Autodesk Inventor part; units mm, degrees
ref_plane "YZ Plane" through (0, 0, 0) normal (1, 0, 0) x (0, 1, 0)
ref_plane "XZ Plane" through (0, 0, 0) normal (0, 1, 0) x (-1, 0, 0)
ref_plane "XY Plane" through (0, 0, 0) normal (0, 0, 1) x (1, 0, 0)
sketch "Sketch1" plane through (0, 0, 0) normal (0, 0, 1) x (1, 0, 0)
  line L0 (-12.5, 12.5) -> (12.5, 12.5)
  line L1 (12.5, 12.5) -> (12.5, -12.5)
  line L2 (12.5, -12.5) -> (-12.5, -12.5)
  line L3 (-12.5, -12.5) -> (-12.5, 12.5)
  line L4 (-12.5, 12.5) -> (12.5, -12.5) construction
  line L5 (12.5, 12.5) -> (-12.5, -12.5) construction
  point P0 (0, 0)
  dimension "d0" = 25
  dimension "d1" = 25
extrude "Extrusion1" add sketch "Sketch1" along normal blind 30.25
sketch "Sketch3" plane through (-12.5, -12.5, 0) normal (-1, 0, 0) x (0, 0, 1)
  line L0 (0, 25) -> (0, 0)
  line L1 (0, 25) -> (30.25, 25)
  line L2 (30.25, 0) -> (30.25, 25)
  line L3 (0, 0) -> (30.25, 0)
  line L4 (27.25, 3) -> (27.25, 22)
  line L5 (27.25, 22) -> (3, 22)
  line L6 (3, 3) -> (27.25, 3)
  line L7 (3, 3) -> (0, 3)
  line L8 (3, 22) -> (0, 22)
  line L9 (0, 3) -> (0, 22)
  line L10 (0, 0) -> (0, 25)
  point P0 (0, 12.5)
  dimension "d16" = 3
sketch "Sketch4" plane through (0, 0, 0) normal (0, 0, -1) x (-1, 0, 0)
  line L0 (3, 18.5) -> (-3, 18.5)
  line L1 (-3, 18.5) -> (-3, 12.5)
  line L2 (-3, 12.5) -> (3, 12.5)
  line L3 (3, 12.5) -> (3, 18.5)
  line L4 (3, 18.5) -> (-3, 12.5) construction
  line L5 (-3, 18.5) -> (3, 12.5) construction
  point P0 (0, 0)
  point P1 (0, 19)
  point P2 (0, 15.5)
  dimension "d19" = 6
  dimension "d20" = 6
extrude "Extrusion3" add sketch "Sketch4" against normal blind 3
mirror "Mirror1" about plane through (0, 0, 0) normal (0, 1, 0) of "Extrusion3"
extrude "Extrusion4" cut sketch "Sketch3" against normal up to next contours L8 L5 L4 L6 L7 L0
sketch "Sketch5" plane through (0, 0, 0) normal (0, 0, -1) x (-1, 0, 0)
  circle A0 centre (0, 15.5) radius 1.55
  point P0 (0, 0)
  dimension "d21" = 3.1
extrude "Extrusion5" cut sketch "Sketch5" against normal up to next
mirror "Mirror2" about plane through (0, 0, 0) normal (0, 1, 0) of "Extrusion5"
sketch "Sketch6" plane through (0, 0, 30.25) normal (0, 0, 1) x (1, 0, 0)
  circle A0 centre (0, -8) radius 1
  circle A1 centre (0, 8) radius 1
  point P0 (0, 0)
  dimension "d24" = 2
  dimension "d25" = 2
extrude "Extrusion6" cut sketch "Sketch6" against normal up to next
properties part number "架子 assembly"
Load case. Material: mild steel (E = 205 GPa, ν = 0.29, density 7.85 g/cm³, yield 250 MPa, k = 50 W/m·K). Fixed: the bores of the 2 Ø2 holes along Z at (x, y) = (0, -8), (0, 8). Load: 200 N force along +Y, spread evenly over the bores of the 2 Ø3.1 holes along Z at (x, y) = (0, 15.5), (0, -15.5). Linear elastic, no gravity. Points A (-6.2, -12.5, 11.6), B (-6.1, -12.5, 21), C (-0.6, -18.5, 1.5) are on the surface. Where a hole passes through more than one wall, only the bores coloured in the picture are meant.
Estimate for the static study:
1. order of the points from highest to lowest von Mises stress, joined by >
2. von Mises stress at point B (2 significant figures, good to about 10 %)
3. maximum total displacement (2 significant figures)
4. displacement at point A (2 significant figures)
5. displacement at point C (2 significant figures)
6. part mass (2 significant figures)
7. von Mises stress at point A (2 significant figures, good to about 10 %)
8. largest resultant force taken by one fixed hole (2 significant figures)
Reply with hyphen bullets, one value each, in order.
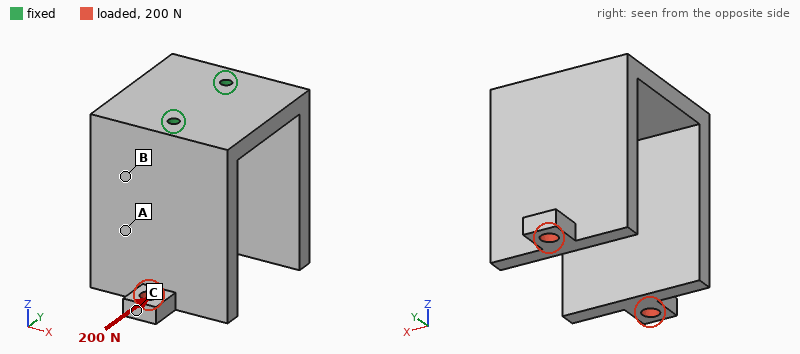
- B > A > C
- 48 MPa
- 90 µm
- 40 µm
- 84 µm
- 48 g
- 27 MPa
- 200 N
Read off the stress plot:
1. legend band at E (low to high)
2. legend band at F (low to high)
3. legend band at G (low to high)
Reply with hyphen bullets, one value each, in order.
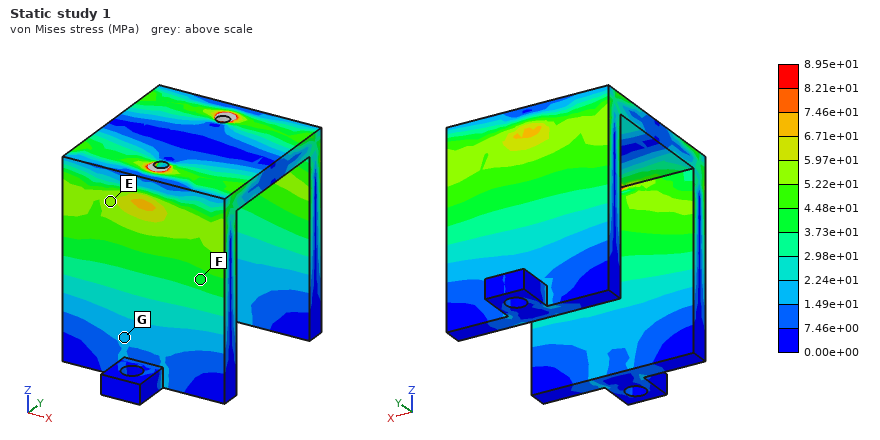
- 5.22e+01 to 5.97e+01 MPa
- 3.73e+01 to 4.48e+01 MPa
- 1.49e+01 to 2.24e+01 MPa
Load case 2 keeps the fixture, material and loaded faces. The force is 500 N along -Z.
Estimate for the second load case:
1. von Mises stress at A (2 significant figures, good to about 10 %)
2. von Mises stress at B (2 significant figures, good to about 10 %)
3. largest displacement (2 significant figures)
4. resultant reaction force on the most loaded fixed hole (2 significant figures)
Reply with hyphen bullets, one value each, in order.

- 33 MPa
- 31 MPa
- 69 µm
- 250 N
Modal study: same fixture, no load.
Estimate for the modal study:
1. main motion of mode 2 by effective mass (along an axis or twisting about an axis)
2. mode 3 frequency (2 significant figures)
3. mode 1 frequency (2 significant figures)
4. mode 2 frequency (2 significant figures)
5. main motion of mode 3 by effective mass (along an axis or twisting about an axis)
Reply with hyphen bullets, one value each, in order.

- along Y
- 3200 Hz
- 2300 Hz
- 2400 Hz
- along X
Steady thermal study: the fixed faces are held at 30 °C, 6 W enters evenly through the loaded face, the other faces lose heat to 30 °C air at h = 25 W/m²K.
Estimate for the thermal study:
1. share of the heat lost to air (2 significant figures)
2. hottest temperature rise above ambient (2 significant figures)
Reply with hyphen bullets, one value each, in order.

- 24 %
- 44 K
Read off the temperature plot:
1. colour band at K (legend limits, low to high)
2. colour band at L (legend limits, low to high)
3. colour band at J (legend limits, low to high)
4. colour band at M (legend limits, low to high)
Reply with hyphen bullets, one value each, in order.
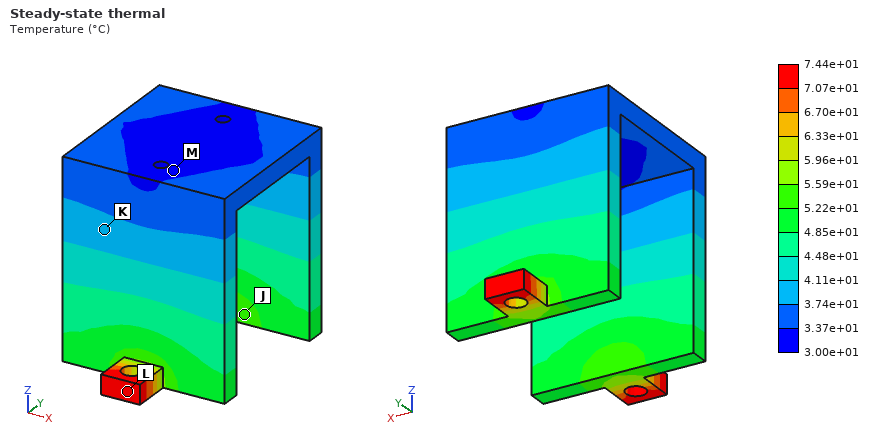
- 3.74e+01 to 4.11e+01 °C
- 7.07e+01 to 7.44e+01 °C
- 5.22e+01 to 5.59e+01 °C
- 3.00e+01 to 3.37e+01 °C
